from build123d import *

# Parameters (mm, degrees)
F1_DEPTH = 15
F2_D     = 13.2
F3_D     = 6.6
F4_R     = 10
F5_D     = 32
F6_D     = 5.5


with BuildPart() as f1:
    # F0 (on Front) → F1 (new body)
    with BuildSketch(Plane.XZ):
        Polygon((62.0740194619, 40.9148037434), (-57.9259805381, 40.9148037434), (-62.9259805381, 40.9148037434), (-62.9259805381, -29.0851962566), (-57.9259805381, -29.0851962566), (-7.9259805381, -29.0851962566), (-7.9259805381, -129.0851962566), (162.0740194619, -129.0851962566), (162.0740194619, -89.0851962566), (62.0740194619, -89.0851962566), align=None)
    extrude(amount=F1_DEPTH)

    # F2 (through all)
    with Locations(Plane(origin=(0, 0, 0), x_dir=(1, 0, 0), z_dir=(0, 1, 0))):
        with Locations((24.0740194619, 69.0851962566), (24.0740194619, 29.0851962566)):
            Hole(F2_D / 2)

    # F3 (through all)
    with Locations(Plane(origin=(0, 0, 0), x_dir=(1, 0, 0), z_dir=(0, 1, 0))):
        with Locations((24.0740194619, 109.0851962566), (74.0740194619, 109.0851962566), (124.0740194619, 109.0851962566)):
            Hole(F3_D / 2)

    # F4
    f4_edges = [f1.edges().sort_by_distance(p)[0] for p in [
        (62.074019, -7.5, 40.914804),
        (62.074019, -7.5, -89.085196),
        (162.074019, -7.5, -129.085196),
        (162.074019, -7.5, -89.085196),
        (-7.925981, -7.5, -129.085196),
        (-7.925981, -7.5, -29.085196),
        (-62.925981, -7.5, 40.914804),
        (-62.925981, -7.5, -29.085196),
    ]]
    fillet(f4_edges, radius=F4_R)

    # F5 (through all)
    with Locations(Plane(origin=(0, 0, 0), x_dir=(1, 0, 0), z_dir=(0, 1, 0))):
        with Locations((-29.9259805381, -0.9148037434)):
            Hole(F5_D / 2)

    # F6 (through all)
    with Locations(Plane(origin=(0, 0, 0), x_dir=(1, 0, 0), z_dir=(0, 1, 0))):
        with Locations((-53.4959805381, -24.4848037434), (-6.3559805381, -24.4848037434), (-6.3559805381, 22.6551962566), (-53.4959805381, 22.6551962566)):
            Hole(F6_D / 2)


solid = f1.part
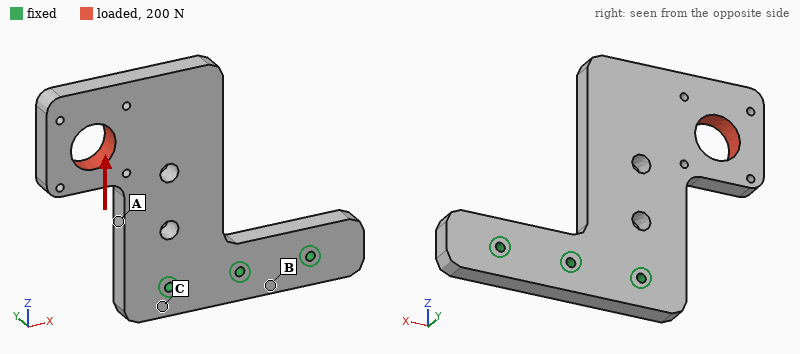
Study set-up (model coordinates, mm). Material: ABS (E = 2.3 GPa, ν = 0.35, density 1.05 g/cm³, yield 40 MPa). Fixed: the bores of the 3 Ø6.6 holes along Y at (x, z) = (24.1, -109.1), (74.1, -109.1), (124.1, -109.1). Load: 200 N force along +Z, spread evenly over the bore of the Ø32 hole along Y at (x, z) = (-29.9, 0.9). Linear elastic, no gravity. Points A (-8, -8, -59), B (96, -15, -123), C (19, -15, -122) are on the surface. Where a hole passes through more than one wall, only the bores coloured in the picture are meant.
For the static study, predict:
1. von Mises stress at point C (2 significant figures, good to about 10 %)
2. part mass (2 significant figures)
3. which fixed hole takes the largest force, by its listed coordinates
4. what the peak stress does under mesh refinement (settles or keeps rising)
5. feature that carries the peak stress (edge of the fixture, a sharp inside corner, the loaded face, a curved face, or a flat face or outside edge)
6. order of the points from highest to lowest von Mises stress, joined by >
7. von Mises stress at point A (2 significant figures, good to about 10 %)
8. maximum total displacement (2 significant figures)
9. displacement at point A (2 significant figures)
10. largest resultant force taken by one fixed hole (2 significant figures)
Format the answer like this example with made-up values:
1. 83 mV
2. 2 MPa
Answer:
1. 0.59 MPa
2. 290 g
3. (24.1, -109.1)
4. keeps rising
5. edge of the fixture
6. A > C > B
7. 1.1 MPa
8. 0.25 mm
9. 0.055 mm
10. 390 N
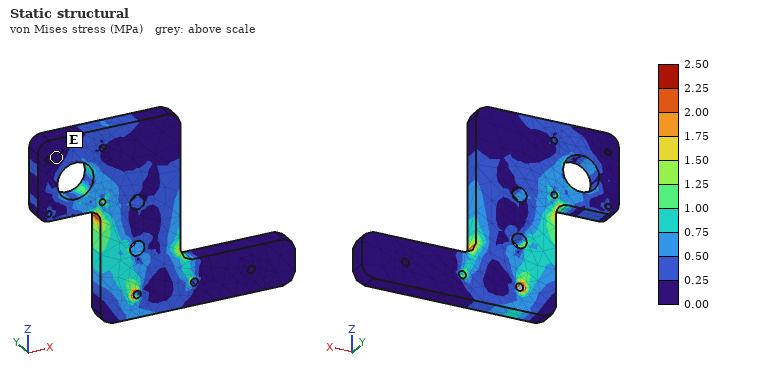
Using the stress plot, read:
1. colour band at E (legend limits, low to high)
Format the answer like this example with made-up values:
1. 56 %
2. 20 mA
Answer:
1. 0.00 to 0.25 MPa
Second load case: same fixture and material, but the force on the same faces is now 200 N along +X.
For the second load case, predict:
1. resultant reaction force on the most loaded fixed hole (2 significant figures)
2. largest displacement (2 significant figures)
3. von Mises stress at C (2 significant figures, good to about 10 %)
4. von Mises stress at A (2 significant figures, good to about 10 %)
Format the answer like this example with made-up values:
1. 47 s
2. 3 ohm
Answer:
1. 410 N
2. 0.29 mm
3. 0.74 MPa
4. 0.94 MPa
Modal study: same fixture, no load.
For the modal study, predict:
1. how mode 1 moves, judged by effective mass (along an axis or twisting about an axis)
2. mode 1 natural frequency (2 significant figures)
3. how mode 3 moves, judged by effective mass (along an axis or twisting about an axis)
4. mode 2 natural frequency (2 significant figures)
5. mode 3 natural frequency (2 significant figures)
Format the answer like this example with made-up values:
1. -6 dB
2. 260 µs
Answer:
1. along Y
2. 110 Hz
3. along X
4. 300 Hz
5. 400 Hz
